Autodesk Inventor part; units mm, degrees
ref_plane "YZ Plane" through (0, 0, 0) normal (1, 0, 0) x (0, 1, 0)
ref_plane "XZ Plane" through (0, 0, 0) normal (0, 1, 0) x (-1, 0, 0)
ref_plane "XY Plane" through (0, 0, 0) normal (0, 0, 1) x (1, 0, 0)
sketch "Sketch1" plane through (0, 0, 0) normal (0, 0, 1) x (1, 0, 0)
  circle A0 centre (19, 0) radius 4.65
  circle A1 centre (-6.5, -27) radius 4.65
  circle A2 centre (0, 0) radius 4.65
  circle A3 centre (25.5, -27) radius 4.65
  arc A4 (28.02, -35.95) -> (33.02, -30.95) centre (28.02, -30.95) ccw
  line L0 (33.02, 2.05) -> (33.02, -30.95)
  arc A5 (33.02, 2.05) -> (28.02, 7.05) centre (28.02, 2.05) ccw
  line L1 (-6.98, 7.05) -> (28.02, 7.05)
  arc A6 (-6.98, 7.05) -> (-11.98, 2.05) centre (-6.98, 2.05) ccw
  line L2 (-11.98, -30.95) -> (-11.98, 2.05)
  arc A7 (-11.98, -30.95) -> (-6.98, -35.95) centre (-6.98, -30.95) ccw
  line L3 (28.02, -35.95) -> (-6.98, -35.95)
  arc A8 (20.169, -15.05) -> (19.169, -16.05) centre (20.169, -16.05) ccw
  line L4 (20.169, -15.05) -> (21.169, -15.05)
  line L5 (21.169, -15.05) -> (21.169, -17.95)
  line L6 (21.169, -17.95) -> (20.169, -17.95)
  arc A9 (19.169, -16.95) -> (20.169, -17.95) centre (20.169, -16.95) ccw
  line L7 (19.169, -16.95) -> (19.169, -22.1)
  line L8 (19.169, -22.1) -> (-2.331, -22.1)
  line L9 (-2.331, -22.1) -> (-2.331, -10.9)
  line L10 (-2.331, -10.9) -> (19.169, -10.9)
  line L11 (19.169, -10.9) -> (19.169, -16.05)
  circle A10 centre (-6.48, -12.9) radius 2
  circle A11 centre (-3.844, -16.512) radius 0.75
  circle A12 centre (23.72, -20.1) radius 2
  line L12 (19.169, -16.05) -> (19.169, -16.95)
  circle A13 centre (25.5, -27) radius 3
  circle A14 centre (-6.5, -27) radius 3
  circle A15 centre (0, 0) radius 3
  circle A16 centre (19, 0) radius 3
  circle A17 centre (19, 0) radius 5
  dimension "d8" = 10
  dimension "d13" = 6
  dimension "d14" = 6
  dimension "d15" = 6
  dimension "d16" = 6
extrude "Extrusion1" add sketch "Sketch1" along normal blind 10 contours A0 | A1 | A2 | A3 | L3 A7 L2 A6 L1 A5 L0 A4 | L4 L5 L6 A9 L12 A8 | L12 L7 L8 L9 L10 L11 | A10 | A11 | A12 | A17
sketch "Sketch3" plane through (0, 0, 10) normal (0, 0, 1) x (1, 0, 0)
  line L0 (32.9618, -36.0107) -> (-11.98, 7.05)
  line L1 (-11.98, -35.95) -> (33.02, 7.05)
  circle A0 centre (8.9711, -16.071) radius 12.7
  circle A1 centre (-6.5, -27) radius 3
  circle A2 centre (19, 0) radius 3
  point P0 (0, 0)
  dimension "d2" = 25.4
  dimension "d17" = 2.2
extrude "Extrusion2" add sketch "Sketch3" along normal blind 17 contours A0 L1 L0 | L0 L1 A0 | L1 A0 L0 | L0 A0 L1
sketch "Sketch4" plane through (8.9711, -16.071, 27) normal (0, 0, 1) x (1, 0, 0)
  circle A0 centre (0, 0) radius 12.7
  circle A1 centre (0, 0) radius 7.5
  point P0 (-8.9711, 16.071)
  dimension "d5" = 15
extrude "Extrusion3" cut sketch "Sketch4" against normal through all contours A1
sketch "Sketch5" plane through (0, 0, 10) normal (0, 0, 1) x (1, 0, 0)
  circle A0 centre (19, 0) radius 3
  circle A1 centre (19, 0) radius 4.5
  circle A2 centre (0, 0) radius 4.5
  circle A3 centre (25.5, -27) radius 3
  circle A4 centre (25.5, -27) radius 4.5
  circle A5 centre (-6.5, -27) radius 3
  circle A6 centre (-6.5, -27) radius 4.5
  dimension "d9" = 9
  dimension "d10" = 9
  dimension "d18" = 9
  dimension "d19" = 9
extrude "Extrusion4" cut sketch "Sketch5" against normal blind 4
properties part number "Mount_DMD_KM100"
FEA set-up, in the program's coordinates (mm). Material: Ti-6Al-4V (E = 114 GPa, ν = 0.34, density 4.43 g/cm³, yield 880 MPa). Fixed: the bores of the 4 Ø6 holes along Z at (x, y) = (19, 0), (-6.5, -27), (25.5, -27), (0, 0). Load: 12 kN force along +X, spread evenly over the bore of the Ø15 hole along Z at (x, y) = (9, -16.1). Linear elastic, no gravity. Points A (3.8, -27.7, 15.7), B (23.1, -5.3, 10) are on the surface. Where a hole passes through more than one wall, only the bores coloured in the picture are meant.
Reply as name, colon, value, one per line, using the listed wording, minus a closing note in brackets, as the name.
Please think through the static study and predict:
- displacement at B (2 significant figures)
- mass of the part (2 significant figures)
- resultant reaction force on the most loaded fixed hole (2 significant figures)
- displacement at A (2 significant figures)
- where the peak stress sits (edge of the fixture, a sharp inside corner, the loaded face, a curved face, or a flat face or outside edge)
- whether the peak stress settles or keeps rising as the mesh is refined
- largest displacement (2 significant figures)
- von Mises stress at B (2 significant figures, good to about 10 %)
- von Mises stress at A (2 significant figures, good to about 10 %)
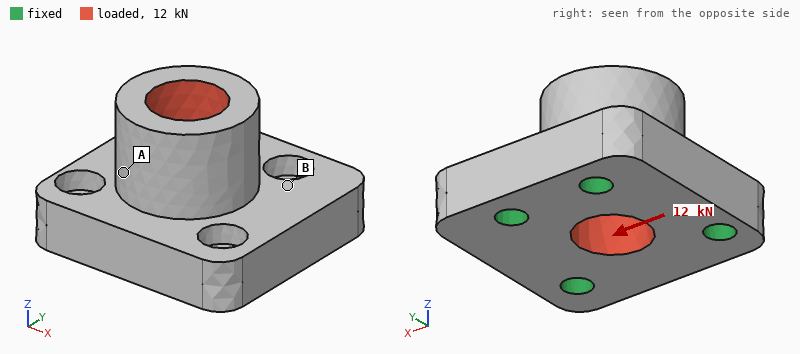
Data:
displacement at B: 4.4 µm
mass of the part: 94 g
resultant reaction force on the most loaded fixed hole: 4.5 kN
displacement at A: 11 µm
where the peak stress sits: edge of the fixture
whether the peak stress settles or keeps rising as the mesh is refined: keeps rising
largest displacement: 23 µm
von Mises stress at B: 15 MPa
von Mises stress at A: 32 MPa
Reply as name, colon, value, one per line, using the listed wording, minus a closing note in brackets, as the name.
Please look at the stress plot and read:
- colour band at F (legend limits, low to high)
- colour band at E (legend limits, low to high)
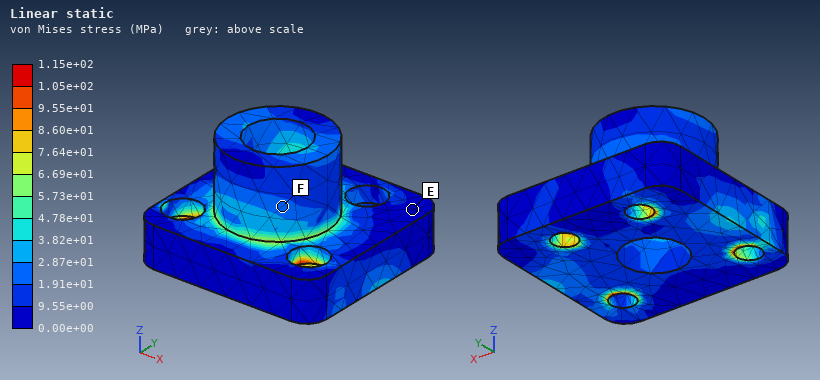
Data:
colour band at F: 1.91e+01 to 2.87e+01 MPa
colour band at E: 0.00e+00 to 9.55e+00 MPa
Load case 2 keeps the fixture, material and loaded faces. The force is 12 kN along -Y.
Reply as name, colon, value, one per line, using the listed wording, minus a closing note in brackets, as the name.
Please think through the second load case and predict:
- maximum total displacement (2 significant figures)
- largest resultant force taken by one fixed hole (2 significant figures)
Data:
maximum total displacement: 25 µm
largest resultant force taken by one fixed hole: 4.1 kN
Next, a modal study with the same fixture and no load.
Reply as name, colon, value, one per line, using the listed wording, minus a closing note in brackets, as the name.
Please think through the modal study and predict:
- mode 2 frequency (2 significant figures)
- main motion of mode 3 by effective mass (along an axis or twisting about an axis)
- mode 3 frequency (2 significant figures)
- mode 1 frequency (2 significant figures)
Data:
mode 2 frequency: 20 kHz
main motion of mode 3 by effective mass: along Z
mode 3 frequency: 28 kHz
mode 1 frequency: 20 kHz
